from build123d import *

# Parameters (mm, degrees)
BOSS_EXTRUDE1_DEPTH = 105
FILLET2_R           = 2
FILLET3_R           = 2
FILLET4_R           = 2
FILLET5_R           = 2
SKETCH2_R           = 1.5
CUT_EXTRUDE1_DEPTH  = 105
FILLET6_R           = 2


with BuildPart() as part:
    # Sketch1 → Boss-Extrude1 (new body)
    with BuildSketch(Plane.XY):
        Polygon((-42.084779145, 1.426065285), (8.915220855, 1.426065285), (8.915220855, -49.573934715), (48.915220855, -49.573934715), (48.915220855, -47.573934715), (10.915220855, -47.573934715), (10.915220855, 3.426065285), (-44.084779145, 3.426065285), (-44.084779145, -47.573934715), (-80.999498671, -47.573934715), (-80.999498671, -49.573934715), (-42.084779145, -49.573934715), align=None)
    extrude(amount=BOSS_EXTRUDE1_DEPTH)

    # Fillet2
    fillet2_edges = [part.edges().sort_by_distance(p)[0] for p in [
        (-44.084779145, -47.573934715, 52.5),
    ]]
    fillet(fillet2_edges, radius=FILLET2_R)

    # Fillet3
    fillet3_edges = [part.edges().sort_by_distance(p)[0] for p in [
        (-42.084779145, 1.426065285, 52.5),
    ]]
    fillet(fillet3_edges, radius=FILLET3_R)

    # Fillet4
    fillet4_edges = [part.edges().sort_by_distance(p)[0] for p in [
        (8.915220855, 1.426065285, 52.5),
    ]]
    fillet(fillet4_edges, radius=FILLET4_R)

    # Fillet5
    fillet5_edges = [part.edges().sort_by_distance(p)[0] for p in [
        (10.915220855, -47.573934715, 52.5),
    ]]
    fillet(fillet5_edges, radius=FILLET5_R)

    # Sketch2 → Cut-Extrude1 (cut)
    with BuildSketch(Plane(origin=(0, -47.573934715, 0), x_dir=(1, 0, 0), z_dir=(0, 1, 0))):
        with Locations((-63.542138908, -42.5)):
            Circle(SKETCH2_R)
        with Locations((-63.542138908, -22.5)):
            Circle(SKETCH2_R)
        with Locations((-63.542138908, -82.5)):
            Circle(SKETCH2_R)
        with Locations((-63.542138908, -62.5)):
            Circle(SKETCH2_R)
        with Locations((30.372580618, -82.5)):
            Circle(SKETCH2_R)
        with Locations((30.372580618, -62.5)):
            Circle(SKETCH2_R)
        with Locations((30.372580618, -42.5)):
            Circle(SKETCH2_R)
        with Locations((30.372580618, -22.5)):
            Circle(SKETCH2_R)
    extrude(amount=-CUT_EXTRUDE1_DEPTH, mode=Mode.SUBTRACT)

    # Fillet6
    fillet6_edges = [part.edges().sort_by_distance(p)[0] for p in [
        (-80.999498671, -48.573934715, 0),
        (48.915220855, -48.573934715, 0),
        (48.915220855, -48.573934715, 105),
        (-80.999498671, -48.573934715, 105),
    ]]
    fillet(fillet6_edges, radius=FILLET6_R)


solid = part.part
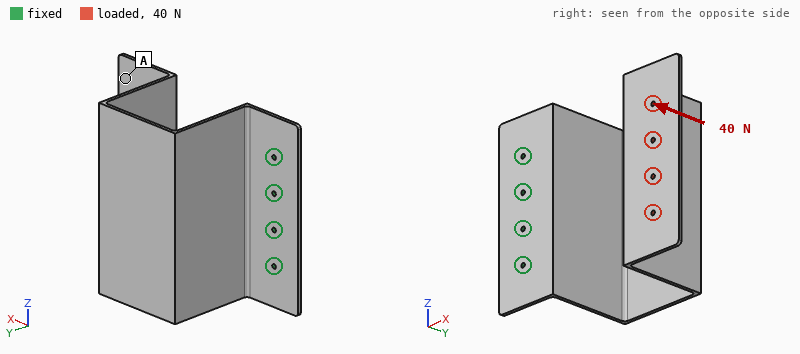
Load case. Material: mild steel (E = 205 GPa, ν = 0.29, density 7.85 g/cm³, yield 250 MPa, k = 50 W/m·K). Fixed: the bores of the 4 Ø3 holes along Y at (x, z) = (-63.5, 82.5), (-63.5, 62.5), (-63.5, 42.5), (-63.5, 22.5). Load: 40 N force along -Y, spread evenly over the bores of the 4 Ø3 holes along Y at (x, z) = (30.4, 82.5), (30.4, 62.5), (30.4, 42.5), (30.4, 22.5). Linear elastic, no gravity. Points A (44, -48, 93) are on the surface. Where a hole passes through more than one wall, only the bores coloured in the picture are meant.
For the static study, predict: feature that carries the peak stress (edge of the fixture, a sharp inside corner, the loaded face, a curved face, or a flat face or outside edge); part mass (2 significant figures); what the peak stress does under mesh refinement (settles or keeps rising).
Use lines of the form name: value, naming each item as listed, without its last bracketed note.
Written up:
feature that carries the peak stress: edge of the fixture
part mass: 380 g
what the peak stress does under mesh refinement: keeps rising
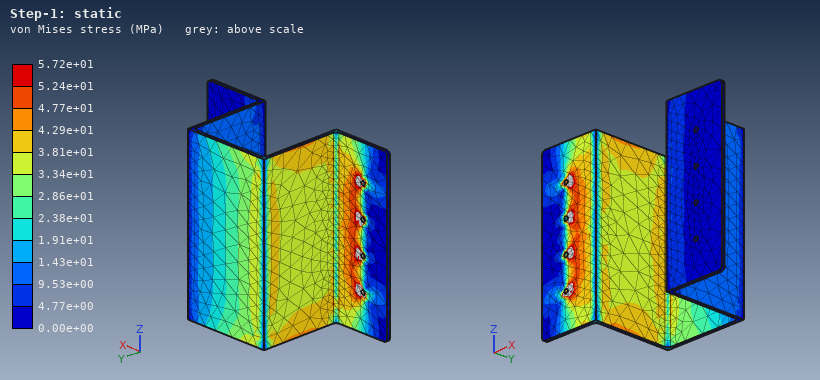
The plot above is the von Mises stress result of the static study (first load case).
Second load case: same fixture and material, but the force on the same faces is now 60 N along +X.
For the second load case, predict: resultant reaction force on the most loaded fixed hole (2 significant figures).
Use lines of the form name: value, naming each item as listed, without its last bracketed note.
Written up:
resultant reaction force on the most loaded fixed hole: 22 N
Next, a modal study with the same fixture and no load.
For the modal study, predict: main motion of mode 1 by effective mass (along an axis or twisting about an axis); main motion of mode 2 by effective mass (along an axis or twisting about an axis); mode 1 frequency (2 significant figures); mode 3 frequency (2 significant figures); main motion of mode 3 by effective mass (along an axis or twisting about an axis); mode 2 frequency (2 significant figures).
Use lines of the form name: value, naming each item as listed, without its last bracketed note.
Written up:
main motion of mode 1 by effective mass: along Y
main motion of mode 2 by effective mass: along Z
mode 1 frequency: 70 Hz
mode 3 frequency: 150 Hz
main motion of mode 3 by effective mass: along X
mode 2 frequency: 130 Hz
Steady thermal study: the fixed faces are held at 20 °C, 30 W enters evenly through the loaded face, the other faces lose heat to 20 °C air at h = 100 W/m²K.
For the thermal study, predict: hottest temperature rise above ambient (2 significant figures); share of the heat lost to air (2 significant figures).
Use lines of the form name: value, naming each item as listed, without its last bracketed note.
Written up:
hottest temperature rise above ambient: 56 K
share of the heat lost to air: 100 %
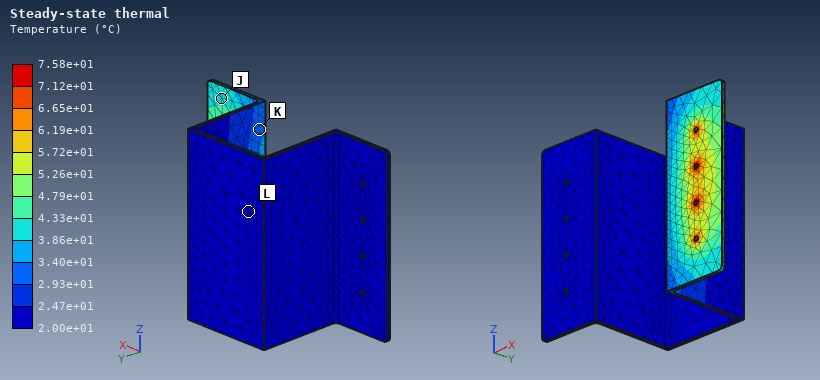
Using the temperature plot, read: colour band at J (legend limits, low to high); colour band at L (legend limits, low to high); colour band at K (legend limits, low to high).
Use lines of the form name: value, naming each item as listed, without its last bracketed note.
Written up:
colour band at J: 3.86e+01 to 4.33e+01 °C
colour band at L: 2.00e+01 to 2.47e+01 °C
colour band at K: 2.93e+01 to 3.40e+01 °C
